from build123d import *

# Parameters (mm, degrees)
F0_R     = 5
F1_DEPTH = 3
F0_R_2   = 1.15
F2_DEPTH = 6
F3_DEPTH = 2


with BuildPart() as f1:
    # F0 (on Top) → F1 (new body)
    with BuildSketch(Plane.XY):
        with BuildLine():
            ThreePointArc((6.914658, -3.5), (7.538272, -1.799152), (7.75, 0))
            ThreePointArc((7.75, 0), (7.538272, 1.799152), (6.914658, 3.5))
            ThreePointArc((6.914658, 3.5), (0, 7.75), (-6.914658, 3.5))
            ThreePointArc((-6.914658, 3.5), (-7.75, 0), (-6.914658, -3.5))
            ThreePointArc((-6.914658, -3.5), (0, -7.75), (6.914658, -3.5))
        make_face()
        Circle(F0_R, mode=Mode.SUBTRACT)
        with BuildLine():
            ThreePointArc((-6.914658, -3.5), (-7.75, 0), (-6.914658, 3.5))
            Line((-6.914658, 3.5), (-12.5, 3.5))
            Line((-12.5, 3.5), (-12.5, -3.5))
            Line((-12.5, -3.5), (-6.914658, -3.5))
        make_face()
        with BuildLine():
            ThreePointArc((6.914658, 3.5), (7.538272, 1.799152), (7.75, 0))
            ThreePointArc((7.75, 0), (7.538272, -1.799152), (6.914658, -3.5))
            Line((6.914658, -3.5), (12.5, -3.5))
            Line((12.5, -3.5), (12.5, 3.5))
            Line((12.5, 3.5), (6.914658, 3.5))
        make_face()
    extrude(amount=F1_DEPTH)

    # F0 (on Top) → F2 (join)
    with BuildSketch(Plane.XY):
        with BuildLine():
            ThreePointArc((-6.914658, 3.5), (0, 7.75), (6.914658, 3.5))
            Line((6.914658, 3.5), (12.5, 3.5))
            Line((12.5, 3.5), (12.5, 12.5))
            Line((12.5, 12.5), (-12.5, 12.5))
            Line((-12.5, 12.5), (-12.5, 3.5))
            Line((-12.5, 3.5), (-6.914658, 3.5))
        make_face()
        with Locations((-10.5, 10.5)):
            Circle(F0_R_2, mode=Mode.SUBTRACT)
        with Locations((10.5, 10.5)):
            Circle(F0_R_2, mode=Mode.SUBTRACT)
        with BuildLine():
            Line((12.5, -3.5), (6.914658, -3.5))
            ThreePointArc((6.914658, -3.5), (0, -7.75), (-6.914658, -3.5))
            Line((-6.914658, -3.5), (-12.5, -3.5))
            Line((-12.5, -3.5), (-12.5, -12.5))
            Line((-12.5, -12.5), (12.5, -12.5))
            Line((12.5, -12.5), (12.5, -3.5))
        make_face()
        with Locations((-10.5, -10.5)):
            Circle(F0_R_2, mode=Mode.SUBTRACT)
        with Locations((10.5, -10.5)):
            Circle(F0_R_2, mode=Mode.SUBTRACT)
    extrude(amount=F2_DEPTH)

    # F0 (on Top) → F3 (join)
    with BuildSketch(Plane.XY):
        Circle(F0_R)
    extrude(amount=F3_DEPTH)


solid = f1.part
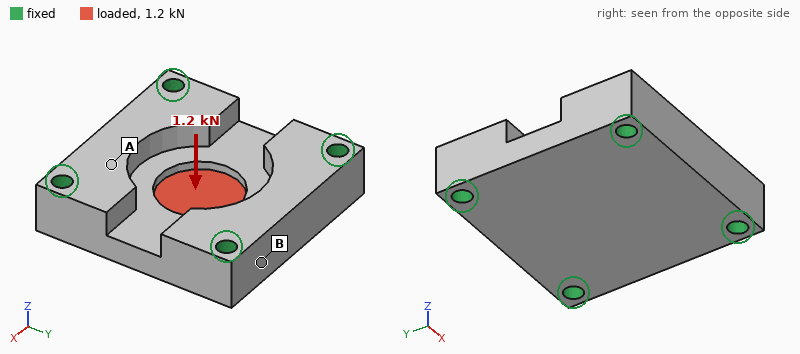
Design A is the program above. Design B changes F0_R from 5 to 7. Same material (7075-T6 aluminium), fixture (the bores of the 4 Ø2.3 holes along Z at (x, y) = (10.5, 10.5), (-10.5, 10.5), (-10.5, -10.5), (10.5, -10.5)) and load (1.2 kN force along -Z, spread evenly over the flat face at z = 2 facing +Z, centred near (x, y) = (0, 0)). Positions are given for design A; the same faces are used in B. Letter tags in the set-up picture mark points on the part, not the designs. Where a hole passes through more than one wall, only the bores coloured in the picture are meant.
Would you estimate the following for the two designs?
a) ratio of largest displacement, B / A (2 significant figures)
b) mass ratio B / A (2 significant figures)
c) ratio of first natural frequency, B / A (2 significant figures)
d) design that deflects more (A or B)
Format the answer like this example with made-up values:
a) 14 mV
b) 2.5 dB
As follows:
a) 0.89
b) 0.97
c) 1.0
d) A
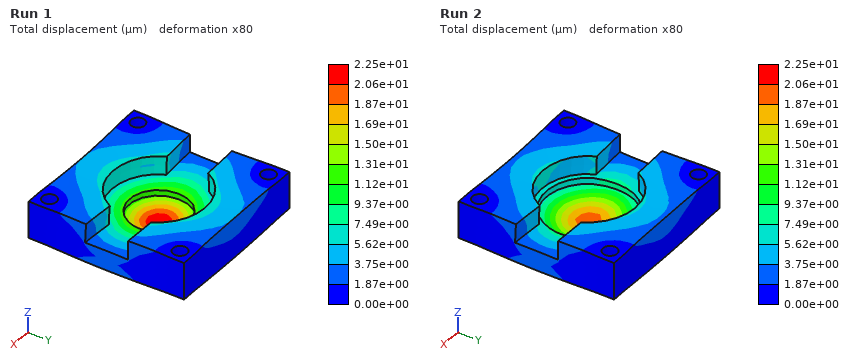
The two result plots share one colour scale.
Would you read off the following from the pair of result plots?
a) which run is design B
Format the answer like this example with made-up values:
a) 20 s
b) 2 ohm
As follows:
a) Run 2
